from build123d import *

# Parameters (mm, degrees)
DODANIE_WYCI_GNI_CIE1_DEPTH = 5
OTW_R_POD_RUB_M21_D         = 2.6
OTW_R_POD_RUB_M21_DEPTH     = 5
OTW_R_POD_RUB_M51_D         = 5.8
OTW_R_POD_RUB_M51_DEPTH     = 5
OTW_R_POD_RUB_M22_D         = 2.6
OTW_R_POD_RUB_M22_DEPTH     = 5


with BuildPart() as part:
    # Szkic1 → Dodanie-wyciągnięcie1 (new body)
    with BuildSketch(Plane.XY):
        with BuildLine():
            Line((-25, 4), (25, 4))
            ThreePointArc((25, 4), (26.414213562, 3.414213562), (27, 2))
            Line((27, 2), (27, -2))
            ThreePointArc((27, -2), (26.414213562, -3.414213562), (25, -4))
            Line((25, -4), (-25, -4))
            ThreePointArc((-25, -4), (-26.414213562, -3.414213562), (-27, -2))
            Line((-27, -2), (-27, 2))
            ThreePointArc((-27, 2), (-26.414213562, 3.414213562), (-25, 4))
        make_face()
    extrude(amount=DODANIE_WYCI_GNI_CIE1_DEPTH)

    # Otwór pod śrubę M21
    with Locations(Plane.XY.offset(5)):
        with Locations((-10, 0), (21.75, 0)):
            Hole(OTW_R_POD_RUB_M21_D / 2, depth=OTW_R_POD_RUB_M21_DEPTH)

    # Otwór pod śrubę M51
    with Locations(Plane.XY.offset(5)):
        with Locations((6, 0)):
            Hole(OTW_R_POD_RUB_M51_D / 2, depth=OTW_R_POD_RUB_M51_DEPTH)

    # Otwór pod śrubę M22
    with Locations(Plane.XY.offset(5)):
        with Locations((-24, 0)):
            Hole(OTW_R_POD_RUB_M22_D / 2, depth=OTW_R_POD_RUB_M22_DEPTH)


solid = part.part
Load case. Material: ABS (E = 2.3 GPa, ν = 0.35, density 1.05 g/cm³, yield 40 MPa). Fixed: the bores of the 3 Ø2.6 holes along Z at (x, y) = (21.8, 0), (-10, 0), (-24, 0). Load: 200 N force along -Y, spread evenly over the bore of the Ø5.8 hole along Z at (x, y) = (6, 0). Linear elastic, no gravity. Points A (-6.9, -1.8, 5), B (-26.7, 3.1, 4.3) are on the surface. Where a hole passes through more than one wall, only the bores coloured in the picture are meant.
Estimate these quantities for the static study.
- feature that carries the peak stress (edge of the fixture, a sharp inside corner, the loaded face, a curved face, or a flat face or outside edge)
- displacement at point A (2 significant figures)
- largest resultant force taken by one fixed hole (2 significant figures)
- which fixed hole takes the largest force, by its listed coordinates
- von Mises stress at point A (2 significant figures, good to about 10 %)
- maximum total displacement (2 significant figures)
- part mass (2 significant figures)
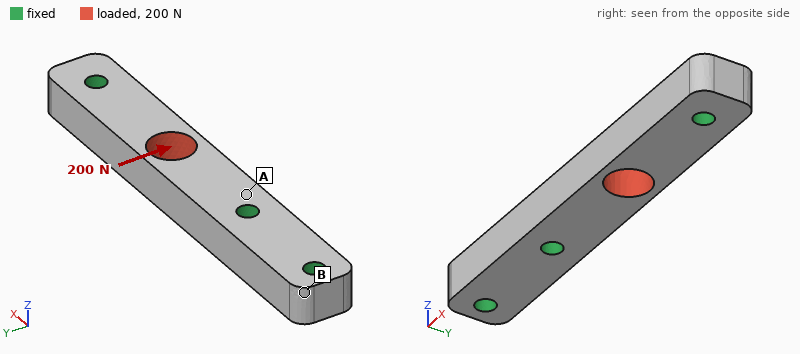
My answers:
edge of the fixture
0.025 mm
130 N
(-10, 0)
6.4 MPa
0.16 mm
2.0 g
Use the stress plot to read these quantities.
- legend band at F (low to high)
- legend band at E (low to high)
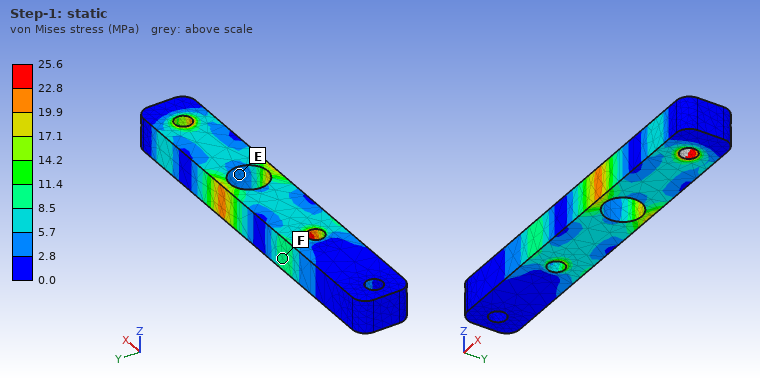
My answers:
8.5 to 11.4 MPa
2.8 to 5.7 MPa
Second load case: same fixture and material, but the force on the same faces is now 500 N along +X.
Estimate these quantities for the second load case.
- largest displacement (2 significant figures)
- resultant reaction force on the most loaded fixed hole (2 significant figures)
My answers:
46 µm
250 N
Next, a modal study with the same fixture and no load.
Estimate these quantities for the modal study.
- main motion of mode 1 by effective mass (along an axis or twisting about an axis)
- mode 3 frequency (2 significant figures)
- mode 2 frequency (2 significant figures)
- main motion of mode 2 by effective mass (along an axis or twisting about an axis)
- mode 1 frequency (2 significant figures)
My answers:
along Z
12 kHz
8500 Hz
along Y
6800 Hz
